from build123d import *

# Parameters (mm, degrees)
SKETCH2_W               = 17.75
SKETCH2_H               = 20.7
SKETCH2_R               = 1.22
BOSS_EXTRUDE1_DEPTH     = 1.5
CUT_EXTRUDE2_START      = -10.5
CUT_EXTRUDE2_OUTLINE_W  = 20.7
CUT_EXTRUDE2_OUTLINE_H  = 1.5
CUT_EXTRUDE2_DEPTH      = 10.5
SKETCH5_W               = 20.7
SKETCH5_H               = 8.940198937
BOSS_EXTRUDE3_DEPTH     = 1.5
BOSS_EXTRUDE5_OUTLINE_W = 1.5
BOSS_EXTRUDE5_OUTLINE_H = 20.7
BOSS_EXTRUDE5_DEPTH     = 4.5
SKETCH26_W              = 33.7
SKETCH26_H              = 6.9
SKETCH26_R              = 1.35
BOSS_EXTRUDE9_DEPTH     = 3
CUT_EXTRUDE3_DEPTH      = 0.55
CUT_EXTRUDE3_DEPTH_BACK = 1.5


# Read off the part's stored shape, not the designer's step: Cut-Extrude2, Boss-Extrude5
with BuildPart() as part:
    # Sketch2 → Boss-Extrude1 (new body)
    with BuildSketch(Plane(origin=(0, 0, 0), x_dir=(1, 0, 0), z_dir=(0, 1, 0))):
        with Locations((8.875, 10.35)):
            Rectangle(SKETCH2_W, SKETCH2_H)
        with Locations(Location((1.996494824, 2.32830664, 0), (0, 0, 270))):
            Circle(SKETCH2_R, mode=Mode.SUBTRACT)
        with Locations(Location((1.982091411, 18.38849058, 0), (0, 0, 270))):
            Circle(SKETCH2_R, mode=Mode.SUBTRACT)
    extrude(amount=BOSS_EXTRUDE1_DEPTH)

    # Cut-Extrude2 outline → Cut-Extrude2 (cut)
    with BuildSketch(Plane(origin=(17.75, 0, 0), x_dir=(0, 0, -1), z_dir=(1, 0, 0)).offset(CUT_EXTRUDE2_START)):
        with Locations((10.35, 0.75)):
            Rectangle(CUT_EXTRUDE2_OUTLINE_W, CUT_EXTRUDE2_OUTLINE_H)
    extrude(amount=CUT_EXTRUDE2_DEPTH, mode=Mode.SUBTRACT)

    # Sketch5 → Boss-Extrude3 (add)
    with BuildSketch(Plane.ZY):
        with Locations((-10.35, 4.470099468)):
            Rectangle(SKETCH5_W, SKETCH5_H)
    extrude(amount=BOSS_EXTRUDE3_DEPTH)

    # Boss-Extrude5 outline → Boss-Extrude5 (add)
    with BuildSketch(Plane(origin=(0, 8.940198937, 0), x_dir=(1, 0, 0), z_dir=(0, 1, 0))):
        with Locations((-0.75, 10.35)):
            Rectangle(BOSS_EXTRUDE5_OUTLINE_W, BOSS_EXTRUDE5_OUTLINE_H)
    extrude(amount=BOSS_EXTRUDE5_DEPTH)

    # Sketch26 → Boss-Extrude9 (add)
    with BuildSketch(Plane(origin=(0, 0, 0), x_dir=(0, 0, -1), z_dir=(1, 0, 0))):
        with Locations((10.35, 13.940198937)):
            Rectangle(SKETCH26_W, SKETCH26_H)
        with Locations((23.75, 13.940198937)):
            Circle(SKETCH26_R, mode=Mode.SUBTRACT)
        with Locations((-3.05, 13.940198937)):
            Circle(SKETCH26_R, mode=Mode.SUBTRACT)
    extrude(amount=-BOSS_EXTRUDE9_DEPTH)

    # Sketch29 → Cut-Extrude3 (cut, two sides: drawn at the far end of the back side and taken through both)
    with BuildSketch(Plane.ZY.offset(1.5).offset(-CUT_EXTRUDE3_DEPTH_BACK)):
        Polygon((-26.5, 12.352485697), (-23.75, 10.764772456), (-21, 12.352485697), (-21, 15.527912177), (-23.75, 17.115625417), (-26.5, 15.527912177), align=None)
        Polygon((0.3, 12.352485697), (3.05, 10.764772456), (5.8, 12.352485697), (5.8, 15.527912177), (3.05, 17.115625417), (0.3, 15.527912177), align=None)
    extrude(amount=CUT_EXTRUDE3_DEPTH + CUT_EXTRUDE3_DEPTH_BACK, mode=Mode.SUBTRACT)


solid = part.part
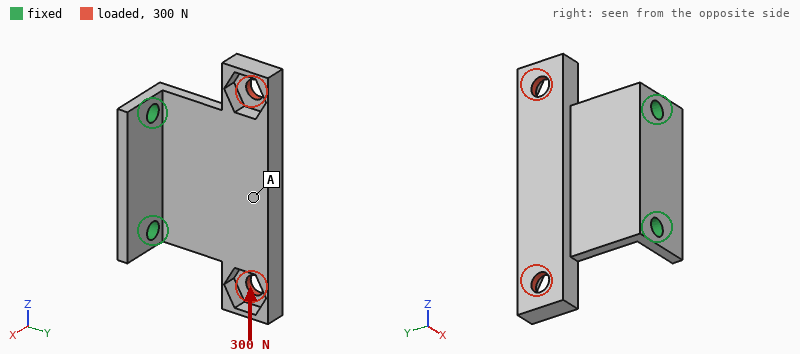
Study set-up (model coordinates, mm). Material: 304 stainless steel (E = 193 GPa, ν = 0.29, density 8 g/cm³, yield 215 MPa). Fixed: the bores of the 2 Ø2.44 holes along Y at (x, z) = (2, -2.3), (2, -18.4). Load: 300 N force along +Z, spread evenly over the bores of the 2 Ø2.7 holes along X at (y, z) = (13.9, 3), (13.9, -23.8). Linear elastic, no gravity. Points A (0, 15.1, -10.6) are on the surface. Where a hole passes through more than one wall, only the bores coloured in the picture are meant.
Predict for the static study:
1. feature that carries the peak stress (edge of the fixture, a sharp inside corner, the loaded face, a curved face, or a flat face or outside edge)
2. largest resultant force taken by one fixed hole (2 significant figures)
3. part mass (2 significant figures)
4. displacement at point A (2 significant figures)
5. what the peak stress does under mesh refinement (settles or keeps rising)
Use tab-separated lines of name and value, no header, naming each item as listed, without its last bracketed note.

feature that carries the peak stress	edge of the fixture
largest resultant force taken by one fixed hole	290 N
part mass	8.9 g
displacement at point A	5.2 µm
what the peak stress does under mesh refinement	keeps rising
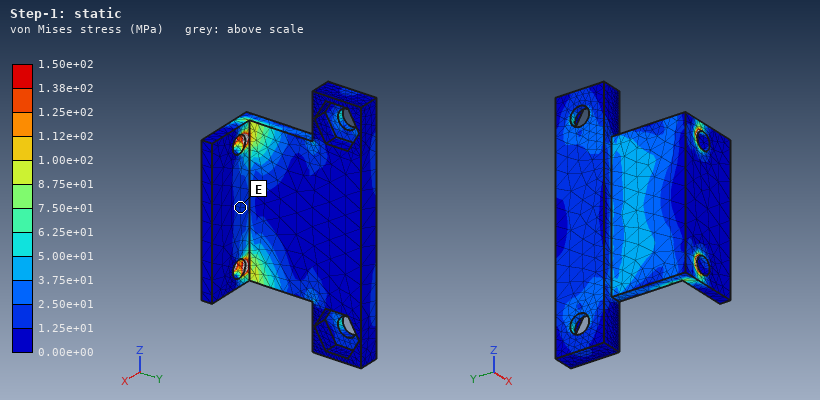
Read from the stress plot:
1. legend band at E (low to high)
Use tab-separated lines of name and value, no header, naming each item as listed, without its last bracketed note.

legend band at E	1.25e+01 to 2.50e+01 MPa
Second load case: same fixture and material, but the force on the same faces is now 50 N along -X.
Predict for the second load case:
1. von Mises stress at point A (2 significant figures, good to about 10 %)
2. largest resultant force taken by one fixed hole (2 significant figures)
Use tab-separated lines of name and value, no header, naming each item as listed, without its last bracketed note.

von Mises stress at point A	12 MPa
largest resultant force taken by one fixed hole	25 N
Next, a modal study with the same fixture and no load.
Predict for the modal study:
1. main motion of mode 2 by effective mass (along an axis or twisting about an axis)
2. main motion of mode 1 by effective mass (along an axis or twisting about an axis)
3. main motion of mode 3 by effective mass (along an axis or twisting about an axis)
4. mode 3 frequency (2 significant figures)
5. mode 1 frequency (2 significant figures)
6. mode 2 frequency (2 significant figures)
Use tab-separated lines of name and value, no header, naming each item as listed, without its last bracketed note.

main motion of mode 2 by effective mass	twisting about Y
main motion of mode 1 by effective mass	along X
main motion of mode 3 by effective mass	along Z
mode 3 frequency	13 kHz
mode 1 frequency	2200 Hz
mode 2 frequency	4900 Hz
